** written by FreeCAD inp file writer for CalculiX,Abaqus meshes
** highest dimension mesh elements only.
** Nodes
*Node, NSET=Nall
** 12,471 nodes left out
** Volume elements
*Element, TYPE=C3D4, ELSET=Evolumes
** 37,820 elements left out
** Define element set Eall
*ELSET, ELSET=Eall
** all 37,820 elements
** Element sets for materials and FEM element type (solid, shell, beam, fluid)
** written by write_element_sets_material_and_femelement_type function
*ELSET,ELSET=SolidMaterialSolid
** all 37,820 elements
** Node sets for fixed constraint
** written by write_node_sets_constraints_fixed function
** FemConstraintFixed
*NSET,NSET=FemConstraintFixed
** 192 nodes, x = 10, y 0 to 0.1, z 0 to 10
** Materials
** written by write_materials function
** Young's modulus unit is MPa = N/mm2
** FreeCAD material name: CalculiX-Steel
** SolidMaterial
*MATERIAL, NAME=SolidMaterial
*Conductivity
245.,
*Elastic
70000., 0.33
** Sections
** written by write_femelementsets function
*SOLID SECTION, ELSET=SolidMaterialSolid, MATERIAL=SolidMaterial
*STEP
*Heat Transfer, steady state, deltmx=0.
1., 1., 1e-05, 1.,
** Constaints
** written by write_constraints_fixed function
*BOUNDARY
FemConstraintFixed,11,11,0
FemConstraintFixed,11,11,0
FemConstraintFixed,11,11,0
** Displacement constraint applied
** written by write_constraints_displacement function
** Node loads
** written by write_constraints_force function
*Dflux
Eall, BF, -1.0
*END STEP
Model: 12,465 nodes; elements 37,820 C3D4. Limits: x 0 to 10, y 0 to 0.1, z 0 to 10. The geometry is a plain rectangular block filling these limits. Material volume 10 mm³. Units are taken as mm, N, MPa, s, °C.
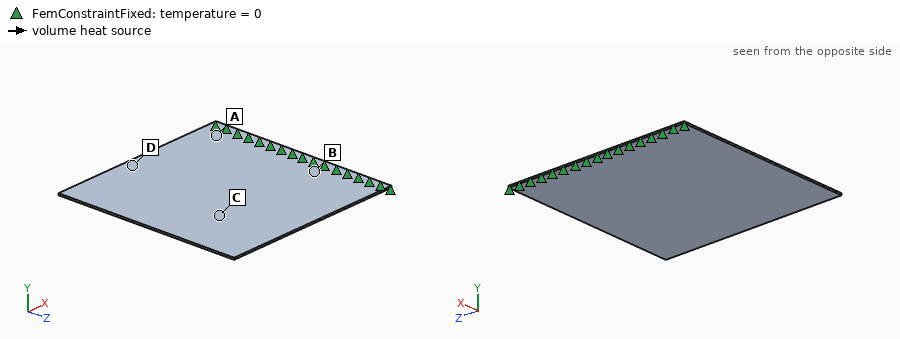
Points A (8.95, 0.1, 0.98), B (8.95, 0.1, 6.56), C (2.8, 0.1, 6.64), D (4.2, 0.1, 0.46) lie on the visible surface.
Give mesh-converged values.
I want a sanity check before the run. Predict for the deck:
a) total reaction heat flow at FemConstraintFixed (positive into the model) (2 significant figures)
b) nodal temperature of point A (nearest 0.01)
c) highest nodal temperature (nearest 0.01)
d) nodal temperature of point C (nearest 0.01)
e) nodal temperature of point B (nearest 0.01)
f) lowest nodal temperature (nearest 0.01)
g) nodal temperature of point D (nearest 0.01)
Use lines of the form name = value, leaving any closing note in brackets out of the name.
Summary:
total reaction heat flow at FemConstraintFixed (positive into the model) = 10 mW
nodal temperature of point A = -0.04 °C
highest nodal temperature = 0.00 °C
nodal temperature of point C = -0.19 °C
nodal temperature of point B = -0.04 °C
lowest nodal temperature = -0.20 °C
nodal temperature of point D = -0.17 °C
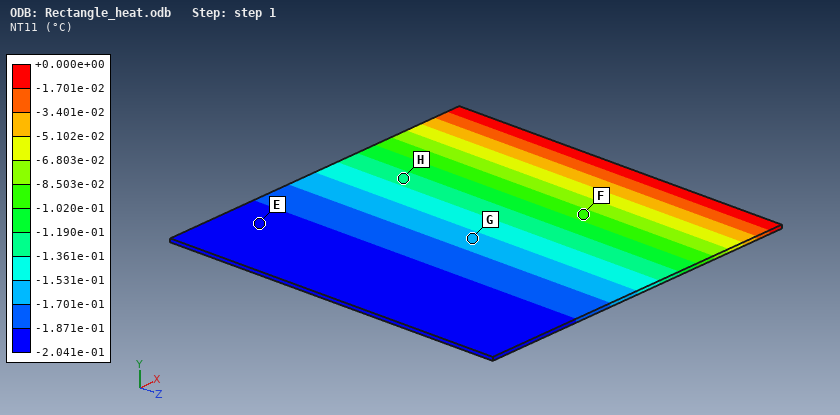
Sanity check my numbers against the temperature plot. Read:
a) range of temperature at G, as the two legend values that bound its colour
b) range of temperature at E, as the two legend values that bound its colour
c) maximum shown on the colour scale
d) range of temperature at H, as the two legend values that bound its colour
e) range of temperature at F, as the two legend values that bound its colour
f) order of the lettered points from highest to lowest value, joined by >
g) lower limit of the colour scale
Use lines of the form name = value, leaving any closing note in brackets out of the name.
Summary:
range of temperature at G, as the two legend values that bound its colour = -1.701e-01 to -1.531e-01 °C
range of temperature at E, as the two legend values that bound its colour = -2.041e-01 to -1.871e-01 °C
maximum shown on the colour scale = +0.000e+00 °C
range of temperature at H, as the two legend values that bound its colour = -1.361e-01 to -1.190e-01 °C
range of temperature at F, as the two legend values that bound its colour = -1.020e-01 to -8.503e-02 °C
order of the lettered points from highest to lowest value, joined by > = F > H > G > E
lower limit of the colour scale = -2.041e-01 °C
